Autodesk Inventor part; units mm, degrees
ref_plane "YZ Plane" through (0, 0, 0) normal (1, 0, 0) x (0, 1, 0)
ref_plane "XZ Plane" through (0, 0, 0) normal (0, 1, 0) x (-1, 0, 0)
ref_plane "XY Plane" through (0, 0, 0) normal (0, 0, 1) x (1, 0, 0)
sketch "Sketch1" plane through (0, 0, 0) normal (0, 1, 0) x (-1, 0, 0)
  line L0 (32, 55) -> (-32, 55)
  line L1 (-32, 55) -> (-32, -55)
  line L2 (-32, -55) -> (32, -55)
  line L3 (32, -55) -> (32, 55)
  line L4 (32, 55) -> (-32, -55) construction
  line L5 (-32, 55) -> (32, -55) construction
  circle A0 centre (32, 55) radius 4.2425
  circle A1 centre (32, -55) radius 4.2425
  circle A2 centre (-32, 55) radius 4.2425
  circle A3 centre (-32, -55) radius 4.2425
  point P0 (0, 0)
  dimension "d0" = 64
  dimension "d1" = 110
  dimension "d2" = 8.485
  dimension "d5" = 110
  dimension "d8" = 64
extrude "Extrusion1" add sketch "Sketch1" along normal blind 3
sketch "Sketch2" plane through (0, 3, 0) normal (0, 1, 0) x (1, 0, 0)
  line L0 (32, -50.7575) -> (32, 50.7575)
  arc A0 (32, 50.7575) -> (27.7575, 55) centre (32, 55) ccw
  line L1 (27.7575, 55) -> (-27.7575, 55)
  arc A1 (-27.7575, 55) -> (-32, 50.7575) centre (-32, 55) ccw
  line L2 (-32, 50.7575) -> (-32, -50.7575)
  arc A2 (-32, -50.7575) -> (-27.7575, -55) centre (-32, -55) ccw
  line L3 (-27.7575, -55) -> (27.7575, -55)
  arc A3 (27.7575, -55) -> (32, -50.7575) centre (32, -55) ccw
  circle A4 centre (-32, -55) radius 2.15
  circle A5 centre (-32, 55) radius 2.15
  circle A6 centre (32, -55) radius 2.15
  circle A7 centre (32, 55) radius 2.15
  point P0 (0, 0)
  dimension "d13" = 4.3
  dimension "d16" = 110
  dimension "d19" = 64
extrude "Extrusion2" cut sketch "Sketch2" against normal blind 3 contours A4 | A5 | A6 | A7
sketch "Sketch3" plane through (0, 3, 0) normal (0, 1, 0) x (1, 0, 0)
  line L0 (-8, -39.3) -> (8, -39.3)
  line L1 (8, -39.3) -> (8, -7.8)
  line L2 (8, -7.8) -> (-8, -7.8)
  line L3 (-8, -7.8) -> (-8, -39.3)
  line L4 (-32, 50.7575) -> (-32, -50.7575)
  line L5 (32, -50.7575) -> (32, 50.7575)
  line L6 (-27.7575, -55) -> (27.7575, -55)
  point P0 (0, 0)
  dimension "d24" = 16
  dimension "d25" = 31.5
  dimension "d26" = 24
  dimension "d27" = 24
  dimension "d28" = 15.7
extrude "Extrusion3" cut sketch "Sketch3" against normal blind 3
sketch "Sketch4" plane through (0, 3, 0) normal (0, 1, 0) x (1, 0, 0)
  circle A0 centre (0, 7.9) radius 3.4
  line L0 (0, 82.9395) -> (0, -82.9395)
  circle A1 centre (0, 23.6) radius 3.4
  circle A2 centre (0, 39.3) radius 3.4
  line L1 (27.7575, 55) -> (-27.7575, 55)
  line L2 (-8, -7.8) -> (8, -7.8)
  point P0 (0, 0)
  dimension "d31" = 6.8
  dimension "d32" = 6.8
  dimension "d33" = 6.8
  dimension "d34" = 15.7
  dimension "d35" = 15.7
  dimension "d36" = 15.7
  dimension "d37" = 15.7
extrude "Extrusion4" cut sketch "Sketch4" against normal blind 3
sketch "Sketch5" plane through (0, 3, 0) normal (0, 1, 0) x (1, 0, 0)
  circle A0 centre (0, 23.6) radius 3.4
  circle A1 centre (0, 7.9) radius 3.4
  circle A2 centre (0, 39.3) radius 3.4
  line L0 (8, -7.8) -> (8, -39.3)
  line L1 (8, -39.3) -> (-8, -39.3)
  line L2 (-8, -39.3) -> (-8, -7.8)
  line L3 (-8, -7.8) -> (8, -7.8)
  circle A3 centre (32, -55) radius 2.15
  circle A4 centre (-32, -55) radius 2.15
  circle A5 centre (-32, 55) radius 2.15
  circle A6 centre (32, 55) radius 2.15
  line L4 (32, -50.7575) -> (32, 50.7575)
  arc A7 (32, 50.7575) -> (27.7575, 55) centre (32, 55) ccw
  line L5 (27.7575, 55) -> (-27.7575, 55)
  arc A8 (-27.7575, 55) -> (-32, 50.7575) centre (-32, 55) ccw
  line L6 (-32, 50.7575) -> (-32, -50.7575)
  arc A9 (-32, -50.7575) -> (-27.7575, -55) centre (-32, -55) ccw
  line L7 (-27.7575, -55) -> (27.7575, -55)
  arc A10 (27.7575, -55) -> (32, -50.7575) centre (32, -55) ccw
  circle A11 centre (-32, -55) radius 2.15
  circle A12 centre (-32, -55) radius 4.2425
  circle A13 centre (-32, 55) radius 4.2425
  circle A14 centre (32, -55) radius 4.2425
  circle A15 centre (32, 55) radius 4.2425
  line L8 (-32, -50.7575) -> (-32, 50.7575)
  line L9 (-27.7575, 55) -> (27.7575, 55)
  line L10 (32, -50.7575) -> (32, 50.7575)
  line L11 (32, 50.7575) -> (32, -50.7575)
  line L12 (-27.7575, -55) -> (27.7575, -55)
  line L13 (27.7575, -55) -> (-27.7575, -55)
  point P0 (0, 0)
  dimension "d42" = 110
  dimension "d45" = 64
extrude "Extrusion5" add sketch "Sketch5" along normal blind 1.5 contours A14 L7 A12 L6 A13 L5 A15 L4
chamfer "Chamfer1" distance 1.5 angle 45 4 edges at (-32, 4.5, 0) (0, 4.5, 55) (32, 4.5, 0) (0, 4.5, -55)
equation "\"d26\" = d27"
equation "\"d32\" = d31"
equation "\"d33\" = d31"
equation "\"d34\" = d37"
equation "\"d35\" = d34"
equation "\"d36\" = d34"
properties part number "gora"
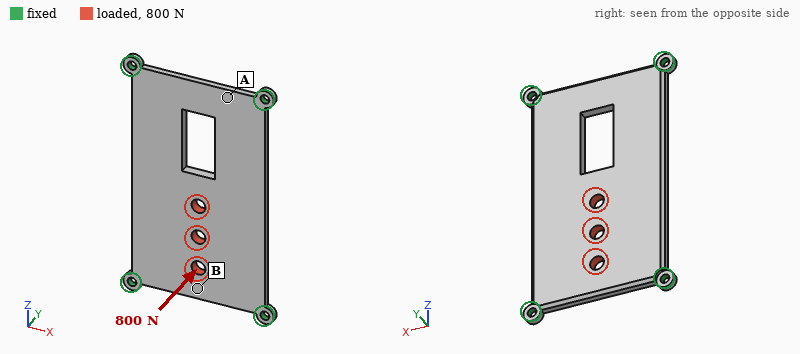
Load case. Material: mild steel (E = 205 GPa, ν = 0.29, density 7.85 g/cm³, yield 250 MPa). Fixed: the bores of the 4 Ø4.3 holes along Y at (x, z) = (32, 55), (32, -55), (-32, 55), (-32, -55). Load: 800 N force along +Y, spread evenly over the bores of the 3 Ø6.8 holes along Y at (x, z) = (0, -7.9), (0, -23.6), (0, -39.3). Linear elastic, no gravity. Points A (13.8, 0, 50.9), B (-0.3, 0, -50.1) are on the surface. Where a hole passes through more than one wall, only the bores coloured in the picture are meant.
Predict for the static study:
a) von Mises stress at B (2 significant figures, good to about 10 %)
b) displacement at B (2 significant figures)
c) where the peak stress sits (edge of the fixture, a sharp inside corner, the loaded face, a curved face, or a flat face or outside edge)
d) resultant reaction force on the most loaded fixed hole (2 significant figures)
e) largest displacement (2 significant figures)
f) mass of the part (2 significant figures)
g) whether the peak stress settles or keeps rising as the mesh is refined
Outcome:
44 MPa
0.036 mm
edge of the fixture
530 N
0.10 mm
230 g
keeps rising
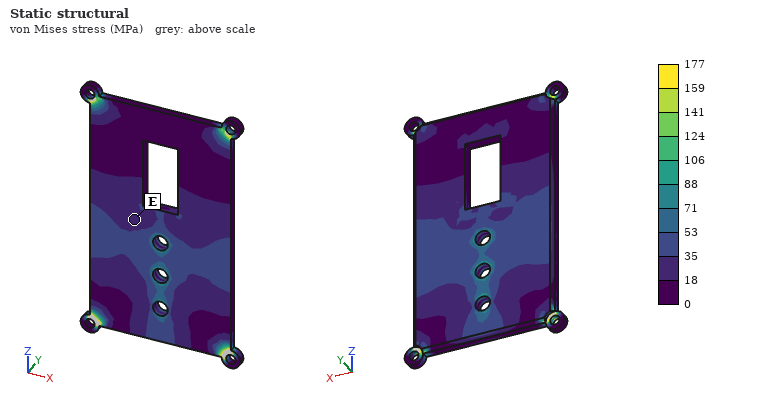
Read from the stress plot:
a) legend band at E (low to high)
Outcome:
18 to 35 MPa
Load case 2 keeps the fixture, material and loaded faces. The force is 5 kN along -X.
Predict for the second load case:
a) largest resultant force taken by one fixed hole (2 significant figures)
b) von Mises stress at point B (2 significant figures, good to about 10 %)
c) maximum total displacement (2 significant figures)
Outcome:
2.3 kN
17 MPa
12 µm
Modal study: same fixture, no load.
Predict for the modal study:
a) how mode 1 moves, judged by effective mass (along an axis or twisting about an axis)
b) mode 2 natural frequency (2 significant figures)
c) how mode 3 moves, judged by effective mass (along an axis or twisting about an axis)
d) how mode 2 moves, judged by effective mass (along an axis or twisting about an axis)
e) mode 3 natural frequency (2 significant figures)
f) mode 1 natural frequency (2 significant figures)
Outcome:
along Y
2500 Hz
twisting about X
twisting about Z
3400 Hz
1200 Hz
